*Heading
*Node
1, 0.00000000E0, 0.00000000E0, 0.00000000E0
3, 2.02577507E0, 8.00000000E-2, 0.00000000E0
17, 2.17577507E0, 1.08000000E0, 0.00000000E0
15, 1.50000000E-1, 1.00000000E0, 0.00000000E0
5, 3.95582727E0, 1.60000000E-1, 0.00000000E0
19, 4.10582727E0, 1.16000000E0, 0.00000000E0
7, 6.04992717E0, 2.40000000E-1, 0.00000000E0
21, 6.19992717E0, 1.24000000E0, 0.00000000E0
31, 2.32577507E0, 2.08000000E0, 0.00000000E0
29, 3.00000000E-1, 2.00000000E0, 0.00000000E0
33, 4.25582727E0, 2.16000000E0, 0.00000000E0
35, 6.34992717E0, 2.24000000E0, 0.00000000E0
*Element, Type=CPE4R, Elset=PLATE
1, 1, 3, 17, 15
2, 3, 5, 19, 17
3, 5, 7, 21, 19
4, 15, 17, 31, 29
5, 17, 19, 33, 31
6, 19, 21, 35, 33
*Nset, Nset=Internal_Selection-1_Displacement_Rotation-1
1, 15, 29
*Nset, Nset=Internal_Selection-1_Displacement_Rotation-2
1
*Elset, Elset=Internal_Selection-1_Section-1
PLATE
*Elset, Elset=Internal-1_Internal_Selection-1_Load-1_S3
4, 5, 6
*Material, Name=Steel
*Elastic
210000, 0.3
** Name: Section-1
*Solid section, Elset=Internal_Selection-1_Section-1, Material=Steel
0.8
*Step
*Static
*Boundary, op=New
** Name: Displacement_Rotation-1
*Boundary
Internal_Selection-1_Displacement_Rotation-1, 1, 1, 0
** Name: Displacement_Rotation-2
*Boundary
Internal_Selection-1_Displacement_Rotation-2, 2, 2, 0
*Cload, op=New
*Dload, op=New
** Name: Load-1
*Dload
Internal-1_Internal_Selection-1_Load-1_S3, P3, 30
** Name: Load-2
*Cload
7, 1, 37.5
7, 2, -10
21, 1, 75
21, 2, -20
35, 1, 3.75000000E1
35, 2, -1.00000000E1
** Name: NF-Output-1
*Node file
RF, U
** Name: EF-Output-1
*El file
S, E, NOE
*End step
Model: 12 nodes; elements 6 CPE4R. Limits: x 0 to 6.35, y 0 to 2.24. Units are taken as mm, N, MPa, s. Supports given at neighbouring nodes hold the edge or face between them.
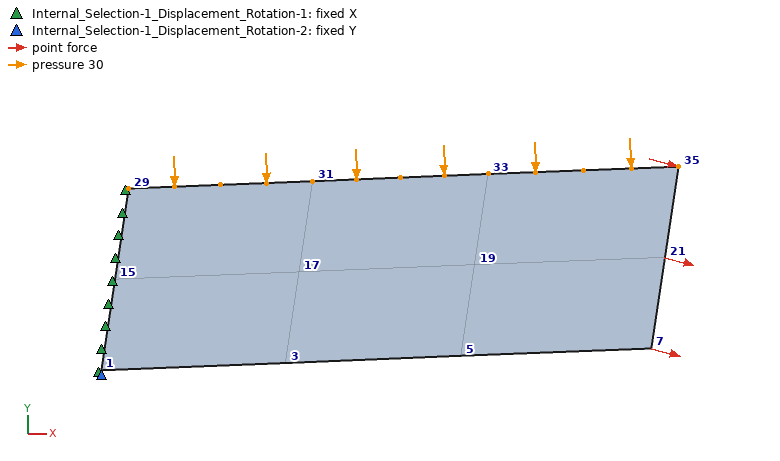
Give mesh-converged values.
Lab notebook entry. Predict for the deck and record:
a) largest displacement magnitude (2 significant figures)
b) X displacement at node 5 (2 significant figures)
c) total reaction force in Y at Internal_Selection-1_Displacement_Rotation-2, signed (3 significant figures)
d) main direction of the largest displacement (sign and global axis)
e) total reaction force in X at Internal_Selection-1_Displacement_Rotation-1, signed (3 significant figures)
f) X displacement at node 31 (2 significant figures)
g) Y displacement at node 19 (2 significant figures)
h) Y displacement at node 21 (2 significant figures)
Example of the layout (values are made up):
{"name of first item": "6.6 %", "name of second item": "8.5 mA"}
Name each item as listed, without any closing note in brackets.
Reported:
{"largest displacement magnitude": "0.080 mm", "X displacement at node 5": "-0.010 mm", "total reaction force in Y at Internal_Selection-1_Displacement_Rotation-2, signed": "185 N", "main direction of the largest displacement": "-Y", "total reaction force in X at Internal_Selection-1_Displacement_Rotation-1, signed": "-156 N", "X displacement at node 31": "0.011 mm", "Y displacement at node 19": "-0.041 mm", "Y displacement at node 21": "-0.073 mm"}
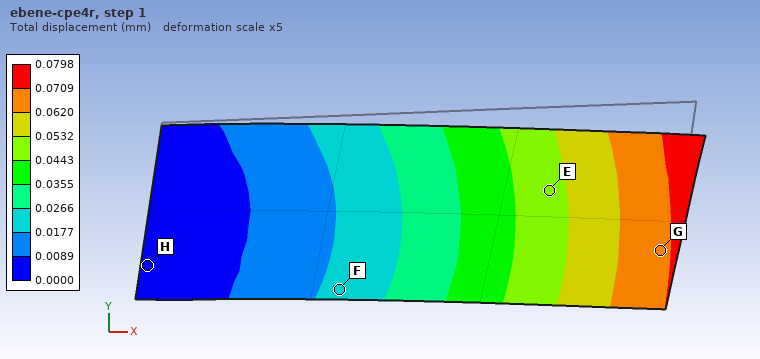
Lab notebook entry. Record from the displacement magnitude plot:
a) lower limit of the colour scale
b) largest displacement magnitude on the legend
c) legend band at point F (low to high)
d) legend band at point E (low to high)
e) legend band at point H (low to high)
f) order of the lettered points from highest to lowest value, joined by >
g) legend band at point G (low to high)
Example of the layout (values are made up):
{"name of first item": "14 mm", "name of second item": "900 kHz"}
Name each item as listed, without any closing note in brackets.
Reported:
{"lower limit of the colour scale": "0.0000 mm", "largest displacement magnitude on the legend": "0.0798 mm", "legend band at point F": "0.0177 to 0.0266 mm", "legend band at point E": "0.0443 to 0.0532 mm", "legend band at point H": "0.0000 to 0.0089 mm", "order of the lettered points from highest to lowest value, joined by >": "G > E > F > H", "legend band at point G": "0.0620 to 0.0709 mm"}
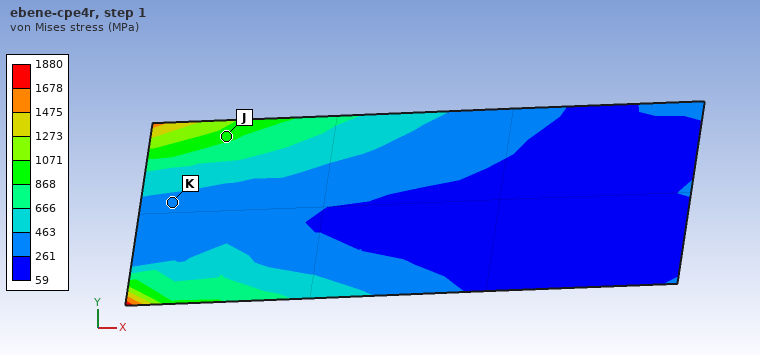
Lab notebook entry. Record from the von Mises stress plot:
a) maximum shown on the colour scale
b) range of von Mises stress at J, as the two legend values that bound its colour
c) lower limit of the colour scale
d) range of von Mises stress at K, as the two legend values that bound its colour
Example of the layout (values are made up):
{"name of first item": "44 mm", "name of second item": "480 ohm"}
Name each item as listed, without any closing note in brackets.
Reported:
{"maximum shown on the colour scale": "1880 MPa", "range of von Mises stress at J, as the two legend values that bound its colour": "868 to 1071 MPa", "lower limit of the colour scale": "59 MPa", "range of von Mises stress at K, as the two legend values that bound its colour": "261 to 463 MPa"}
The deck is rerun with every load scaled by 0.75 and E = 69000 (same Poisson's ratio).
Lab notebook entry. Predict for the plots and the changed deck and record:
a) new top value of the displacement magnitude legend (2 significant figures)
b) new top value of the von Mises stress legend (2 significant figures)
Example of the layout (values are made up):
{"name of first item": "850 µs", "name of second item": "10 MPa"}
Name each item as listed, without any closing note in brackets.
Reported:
{"new top value of the displacement magnitude legend": "0.18 mm", "new top value of the von Mises stress legend": "1400 MPa"}
